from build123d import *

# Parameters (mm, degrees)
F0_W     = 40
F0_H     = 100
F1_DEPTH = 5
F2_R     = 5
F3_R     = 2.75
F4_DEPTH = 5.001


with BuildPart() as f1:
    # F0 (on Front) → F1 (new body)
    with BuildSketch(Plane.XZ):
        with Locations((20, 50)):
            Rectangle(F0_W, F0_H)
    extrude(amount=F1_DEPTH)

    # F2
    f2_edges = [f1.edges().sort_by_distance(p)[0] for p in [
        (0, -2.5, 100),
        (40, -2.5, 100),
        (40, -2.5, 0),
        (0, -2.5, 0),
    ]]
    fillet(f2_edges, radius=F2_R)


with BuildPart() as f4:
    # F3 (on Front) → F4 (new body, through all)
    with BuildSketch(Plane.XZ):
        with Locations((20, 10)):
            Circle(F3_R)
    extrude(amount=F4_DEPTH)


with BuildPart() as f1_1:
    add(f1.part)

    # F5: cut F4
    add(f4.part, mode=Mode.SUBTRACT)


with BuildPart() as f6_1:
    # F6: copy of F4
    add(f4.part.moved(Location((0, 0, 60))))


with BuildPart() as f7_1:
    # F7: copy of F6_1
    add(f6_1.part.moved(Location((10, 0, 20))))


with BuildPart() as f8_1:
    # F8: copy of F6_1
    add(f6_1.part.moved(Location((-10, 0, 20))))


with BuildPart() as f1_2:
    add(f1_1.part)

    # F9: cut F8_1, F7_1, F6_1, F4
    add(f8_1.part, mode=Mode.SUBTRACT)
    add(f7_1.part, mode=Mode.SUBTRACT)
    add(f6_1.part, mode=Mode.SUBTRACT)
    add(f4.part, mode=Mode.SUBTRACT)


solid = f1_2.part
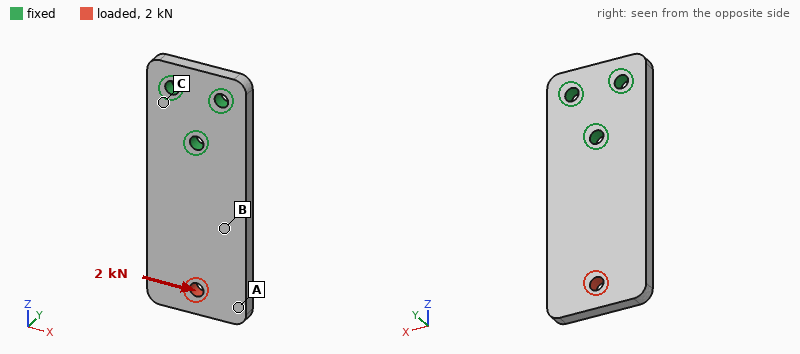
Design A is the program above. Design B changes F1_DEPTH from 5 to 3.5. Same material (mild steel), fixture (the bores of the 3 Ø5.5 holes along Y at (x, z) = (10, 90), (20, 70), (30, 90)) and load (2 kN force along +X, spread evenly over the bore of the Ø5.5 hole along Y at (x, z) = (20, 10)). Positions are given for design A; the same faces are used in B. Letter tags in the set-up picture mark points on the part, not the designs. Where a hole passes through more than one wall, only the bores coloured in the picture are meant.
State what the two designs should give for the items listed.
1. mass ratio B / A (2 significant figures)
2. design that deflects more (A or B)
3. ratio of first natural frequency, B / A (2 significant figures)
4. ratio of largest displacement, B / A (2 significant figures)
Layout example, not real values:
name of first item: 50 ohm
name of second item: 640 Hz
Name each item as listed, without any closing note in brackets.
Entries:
mass ratio B / A: 0.70
design that deflects more: B
ratio of first natural frequency, B / A: 0.71
ratio of largest displacement, B / A: 1.4
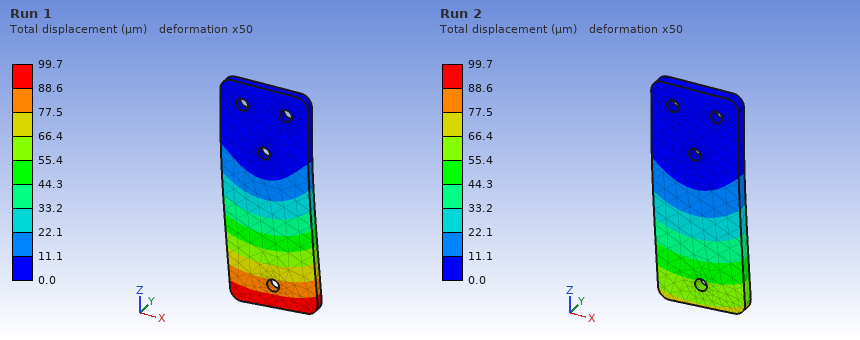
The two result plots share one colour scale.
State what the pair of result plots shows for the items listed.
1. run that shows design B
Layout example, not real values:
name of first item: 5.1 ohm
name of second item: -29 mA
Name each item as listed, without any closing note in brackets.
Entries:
run that shows design B: Run 1
